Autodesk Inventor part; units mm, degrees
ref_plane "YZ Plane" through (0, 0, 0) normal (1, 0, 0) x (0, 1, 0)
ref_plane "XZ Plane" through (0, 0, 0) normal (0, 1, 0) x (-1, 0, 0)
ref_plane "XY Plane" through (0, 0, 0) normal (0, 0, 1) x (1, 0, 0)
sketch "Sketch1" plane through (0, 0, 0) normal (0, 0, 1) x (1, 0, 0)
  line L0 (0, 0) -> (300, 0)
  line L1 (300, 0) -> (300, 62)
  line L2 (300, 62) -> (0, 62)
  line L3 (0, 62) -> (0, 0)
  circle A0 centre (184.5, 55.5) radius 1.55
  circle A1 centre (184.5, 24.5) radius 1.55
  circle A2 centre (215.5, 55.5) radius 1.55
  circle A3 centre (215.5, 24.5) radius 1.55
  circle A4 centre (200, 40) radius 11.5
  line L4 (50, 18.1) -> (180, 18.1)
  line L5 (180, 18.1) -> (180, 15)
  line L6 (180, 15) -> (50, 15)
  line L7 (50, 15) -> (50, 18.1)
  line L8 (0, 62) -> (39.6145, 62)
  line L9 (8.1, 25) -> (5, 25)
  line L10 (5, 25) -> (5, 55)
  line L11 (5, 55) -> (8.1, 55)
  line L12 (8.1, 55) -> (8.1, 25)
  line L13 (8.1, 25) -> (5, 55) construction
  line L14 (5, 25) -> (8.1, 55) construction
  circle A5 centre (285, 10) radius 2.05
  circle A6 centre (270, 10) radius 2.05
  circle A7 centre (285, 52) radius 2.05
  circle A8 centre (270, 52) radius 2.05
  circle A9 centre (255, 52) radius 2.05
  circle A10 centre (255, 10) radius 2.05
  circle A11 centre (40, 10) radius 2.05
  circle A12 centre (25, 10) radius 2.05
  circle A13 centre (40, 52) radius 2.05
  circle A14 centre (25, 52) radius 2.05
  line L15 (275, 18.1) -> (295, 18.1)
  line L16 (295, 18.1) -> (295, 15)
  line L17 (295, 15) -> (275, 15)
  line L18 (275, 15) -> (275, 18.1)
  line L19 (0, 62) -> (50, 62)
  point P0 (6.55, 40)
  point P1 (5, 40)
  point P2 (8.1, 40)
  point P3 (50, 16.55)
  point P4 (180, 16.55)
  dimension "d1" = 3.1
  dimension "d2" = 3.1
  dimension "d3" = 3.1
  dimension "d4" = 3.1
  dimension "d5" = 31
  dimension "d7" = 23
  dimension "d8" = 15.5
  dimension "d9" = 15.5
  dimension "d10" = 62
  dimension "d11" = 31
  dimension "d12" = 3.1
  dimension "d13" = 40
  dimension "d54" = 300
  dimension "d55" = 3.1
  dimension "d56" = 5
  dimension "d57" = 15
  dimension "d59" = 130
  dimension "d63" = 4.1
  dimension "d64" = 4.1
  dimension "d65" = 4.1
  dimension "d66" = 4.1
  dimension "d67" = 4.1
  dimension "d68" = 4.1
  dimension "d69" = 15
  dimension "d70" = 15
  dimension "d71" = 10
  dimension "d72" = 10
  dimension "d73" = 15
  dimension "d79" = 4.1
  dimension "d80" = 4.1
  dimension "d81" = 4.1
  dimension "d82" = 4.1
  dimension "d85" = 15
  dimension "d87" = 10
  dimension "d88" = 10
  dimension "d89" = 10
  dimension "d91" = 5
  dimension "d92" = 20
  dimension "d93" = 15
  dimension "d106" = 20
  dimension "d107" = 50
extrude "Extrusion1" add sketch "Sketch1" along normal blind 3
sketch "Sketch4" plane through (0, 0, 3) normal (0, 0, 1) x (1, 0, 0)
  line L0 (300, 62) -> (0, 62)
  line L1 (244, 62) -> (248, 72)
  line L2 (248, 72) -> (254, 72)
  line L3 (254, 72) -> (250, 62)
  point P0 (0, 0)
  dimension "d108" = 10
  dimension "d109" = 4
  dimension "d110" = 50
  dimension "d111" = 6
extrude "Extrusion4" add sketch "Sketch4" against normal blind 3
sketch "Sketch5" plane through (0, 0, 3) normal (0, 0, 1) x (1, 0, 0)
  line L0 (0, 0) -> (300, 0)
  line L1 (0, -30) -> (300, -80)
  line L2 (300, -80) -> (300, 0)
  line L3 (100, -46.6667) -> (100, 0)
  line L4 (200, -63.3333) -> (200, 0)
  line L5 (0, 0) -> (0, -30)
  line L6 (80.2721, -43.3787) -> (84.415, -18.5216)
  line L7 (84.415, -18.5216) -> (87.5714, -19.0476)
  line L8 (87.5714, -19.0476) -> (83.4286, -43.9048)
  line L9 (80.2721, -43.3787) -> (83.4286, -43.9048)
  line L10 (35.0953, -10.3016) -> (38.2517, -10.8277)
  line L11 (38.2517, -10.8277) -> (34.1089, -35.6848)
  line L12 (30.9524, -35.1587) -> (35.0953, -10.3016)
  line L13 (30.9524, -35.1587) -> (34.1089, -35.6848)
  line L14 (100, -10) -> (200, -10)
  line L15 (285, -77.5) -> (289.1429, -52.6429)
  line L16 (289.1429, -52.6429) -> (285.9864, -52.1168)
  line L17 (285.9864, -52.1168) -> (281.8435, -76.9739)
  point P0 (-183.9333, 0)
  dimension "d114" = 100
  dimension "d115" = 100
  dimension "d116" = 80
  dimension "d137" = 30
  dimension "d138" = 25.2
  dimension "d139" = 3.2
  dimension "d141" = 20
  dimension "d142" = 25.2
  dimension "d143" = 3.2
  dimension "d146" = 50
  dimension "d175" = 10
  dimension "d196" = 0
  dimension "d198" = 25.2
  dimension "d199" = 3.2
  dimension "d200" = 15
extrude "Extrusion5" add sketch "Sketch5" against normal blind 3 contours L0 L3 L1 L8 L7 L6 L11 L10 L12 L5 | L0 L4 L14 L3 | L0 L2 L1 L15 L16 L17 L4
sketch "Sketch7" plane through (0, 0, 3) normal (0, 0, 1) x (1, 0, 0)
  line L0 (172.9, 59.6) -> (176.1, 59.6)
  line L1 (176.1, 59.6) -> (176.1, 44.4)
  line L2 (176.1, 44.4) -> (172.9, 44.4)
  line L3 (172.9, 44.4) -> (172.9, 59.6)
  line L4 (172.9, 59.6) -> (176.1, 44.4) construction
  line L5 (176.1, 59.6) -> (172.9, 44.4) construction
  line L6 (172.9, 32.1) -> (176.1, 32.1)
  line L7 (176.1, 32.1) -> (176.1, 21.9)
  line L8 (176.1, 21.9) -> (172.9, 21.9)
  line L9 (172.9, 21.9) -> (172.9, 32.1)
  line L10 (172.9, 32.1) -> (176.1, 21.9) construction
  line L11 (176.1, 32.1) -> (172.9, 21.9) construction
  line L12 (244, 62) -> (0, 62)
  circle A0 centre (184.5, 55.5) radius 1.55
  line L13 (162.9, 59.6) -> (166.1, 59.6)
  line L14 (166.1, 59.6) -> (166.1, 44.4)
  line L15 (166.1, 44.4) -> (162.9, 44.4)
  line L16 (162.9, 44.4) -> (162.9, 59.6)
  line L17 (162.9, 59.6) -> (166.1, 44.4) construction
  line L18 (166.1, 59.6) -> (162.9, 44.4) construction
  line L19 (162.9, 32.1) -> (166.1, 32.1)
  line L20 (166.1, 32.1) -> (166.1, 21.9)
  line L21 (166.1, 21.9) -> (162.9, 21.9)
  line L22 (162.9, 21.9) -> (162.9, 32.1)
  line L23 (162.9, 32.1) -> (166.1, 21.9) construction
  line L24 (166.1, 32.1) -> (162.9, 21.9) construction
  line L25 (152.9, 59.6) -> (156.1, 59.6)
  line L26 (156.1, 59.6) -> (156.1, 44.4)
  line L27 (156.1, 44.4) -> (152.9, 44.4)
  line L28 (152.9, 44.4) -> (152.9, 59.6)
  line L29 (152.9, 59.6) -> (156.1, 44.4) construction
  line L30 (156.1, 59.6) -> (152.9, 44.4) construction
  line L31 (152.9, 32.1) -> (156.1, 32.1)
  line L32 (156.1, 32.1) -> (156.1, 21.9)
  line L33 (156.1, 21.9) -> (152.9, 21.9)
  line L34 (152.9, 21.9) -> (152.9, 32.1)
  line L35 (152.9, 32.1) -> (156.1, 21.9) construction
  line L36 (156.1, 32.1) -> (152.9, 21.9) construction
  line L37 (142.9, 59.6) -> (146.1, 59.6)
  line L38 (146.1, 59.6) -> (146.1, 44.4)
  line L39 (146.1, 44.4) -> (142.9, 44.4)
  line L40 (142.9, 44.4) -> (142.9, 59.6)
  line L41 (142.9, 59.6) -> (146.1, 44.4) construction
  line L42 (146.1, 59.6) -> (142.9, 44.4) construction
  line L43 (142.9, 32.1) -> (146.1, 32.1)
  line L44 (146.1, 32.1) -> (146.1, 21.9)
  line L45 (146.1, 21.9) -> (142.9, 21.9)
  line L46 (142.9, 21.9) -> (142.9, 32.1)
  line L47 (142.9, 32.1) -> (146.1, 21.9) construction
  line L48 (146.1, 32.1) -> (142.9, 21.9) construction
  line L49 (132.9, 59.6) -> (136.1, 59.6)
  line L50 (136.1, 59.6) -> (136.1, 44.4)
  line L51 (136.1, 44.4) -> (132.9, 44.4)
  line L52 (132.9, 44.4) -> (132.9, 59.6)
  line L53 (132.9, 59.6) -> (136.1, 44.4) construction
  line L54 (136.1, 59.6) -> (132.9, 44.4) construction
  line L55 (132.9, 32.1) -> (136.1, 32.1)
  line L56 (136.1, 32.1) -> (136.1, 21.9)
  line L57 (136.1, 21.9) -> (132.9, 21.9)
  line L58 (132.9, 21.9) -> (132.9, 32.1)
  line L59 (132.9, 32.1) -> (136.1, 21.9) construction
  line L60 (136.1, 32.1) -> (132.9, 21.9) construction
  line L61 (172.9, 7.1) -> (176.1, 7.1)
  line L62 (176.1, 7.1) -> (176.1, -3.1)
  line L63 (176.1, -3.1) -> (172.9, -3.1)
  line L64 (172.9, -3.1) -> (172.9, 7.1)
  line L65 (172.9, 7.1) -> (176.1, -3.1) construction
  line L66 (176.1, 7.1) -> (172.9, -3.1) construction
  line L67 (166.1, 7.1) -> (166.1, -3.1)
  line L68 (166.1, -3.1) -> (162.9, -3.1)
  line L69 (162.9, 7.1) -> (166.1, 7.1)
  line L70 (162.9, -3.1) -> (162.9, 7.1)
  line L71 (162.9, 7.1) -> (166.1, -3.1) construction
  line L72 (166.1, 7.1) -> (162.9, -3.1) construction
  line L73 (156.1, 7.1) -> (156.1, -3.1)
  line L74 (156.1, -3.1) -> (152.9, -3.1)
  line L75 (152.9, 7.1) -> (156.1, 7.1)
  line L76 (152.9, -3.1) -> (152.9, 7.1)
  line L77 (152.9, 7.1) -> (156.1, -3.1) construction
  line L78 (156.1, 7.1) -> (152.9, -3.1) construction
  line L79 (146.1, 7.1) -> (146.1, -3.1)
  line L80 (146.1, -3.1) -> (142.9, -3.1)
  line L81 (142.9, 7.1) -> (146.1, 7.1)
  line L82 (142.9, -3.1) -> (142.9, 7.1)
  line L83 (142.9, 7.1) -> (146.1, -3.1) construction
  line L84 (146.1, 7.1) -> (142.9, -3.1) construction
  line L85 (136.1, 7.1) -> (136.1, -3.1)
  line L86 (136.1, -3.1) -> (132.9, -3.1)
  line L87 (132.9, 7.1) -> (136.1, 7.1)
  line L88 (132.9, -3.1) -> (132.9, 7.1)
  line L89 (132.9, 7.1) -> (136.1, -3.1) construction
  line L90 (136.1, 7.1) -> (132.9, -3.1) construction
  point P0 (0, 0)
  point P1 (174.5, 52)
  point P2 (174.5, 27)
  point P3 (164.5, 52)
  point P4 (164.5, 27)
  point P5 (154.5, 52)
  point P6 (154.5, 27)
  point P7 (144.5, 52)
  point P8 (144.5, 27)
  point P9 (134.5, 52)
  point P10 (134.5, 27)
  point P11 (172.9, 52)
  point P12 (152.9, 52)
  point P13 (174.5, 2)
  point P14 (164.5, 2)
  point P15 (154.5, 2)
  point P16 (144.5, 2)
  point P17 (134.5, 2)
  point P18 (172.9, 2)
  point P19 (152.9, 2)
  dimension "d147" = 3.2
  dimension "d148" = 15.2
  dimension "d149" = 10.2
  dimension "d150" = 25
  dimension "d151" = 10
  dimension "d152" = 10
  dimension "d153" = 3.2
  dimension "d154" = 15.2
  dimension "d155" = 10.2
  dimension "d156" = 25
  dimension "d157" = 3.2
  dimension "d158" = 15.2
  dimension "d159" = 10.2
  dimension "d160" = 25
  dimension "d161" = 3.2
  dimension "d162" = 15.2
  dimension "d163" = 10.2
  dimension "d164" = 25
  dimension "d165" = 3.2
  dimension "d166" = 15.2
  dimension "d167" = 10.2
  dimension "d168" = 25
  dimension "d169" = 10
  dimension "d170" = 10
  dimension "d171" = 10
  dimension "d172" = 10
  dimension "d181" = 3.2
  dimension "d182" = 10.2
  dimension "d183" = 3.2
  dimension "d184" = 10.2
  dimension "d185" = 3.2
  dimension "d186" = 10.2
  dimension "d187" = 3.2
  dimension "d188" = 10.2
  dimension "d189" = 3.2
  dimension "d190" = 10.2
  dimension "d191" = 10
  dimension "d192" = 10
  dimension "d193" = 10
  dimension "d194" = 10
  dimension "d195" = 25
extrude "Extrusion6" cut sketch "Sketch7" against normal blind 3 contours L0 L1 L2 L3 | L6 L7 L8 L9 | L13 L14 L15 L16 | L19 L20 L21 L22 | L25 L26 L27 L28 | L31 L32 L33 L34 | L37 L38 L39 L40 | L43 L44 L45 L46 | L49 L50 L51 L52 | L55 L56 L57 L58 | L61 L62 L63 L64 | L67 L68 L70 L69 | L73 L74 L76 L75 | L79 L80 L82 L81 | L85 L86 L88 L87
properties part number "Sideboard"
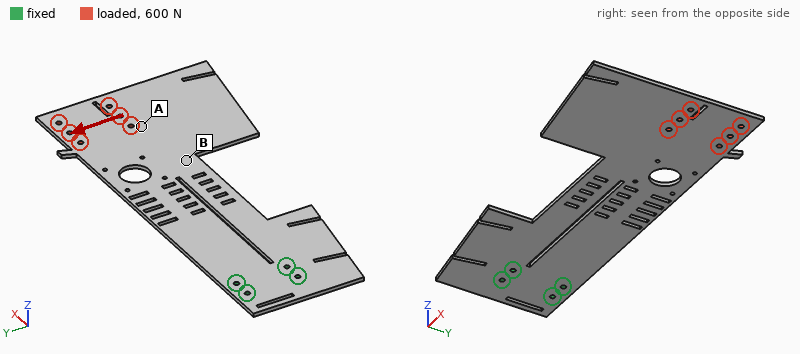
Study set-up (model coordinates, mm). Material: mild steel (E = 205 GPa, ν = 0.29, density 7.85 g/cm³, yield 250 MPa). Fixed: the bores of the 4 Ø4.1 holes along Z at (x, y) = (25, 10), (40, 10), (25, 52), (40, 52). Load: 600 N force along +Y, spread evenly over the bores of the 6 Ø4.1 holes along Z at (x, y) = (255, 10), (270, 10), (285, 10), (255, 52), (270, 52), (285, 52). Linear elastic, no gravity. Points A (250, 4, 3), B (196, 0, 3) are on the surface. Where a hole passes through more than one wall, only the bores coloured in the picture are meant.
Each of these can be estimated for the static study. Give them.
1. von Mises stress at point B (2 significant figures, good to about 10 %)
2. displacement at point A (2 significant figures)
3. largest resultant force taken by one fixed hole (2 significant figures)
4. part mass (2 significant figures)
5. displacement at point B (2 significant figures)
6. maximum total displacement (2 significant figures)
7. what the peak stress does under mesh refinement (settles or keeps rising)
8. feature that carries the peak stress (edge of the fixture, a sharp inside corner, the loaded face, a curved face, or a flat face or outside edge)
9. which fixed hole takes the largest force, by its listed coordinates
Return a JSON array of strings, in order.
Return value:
["15 MPa", "0.18 mm", "2.2 kN", "680 g", "0.12 mm", "0.26 mm", "keeps rising", "edge of the fixture", "(40, 52)"]
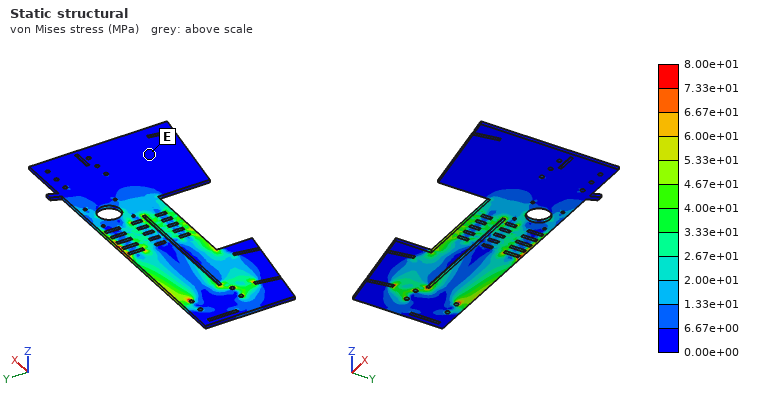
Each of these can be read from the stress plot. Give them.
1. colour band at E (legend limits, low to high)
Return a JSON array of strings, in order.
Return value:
["0.00e+00 to 6.67e+00 MPa"]
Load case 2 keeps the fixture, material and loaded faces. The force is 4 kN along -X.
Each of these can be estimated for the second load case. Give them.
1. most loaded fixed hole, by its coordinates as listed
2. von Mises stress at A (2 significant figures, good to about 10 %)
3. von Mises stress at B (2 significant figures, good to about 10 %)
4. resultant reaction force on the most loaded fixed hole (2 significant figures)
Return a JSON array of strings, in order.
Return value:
["(40, 52)", "17 MPa", "10 MPa", "1.5 kN"]
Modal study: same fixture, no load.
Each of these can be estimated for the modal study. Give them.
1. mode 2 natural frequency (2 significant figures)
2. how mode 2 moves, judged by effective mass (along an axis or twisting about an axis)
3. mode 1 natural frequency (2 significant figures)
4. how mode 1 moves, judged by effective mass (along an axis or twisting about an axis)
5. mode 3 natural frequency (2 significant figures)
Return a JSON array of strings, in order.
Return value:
["110 Hz", "twisting about X", "26 Hz", "along Z", "190 Hz"]
